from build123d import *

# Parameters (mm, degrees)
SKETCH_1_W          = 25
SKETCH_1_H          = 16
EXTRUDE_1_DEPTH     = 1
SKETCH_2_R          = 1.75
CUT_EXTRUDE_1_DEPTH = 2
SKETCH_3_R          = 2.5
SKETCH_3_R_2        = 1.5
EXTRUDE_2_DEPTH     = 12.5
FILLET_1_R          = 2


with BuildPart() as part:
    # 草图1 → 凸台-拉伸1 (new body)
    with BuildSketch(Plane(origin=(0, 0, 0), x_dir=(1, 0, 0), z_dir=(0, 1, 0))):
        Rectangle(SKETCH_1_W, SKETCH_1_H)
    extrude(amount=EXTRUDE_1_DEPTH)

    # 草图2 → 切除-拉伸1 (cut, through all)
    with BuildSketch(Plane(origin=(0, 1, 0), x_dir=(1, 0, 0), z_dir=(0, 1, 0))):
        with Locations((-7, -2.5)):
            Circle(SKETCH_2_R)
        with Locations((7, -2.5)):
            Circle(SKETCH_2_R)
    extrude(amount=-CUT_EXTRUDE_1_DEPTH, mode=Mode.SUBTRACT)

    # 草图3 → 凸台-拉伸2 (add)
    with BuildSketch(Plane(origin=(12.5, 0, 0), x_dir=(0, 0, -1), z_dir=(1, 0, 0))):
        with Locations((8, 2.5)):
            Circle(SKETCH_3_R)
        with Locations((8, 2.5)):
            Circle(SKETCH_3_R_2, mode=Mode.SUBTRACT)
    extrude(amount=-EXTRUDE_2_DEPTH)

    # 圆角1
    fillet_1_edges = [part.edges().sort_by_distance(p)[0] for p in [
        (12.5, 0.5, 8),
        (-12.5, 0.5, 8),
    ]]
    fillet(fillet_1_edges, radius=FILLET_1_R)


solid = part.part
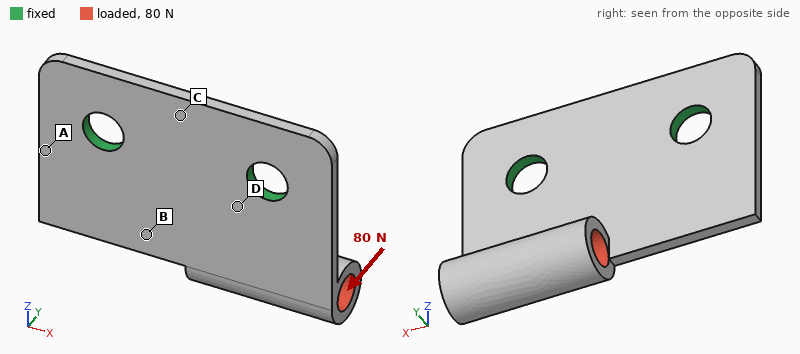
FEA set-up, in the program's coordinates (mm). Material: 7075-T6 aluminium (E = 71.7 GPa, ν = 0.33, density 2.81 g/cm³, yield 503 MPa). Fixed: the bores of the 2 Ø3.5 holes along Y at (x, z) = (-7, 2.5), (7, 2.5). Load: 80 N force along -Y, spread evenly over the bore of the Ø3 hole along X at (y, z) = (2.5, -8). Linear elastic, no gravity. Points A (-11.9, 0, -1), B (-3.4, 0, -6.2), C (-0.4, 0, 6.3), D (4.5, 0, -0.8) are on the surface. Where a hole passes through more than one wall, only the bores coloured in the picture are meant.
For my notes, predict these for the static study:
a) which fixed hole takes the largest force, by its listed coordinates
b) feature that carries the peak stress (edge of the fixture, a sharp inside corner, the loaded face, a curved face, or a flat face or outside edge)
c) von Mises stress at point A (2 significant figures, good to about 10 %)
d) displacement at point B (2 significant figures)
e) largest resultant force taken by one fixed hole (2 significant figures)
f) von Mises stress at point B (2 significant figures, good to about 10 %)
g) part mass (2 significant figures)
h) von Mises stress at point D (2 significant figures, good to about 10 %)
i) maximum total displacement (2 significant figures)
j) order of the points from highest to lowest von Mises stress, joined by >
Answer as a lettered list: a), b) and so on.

a) (7, 2.5)
b) a flat face or outside edge
c) 57 MPa
d) 0.093 mm
e) 69 N
f) 93 MPa
g) 1.5 g
h) 170 MPa
i) 0.31 mm
j) D > B > A > C
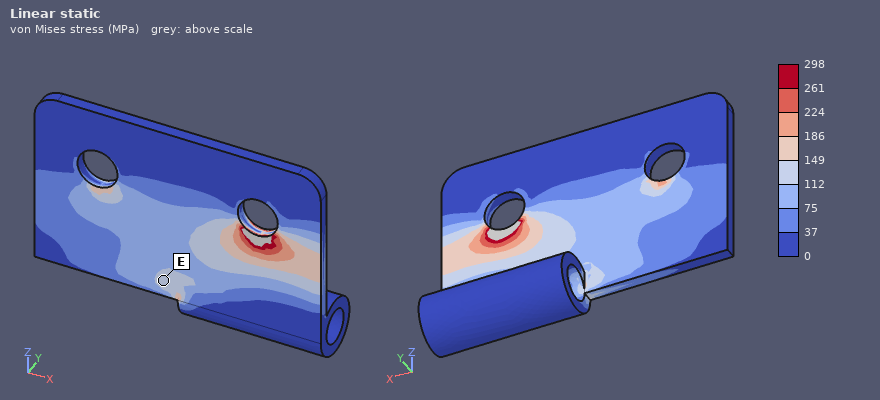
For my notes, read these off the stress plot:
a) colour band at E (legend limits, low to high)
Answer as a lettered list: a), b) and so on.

a) 112 to 149 MPa
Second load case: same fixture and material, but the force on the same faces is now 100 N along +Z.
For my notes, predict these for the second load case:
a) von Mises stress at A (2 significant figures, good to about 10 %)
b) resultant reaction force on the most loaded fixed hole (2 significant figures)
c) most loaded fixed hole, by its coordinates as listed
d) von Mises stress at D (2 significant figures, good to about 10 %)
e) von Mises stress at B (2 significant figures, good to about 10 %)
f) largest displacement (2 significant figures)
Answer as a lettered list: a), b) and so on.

a) 22 MPa
b) 90 N
c) (7, 2.5)
d) 49 MPa
e) 45 MPa
f) 0.12 mm
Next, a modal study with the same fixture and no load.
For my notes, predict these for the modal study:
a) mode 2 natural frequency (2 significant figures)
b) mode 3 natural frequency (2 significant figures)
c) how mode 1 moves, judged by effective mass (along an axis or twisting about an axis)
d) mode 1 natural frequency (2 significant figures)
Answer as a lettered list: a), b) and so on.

a) 9400 Hz
b) 14 kHz
c) along Y
d) 4100 Hz
